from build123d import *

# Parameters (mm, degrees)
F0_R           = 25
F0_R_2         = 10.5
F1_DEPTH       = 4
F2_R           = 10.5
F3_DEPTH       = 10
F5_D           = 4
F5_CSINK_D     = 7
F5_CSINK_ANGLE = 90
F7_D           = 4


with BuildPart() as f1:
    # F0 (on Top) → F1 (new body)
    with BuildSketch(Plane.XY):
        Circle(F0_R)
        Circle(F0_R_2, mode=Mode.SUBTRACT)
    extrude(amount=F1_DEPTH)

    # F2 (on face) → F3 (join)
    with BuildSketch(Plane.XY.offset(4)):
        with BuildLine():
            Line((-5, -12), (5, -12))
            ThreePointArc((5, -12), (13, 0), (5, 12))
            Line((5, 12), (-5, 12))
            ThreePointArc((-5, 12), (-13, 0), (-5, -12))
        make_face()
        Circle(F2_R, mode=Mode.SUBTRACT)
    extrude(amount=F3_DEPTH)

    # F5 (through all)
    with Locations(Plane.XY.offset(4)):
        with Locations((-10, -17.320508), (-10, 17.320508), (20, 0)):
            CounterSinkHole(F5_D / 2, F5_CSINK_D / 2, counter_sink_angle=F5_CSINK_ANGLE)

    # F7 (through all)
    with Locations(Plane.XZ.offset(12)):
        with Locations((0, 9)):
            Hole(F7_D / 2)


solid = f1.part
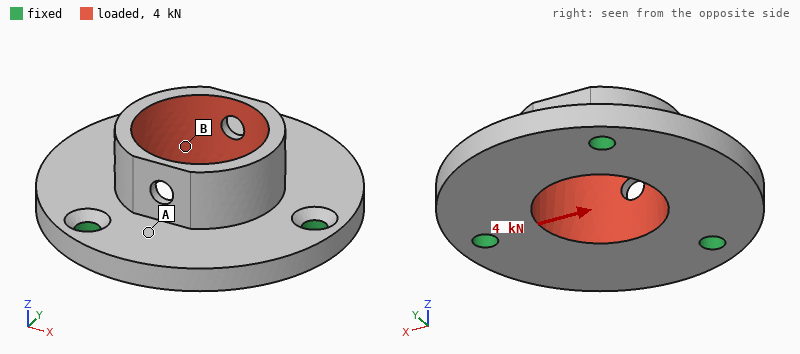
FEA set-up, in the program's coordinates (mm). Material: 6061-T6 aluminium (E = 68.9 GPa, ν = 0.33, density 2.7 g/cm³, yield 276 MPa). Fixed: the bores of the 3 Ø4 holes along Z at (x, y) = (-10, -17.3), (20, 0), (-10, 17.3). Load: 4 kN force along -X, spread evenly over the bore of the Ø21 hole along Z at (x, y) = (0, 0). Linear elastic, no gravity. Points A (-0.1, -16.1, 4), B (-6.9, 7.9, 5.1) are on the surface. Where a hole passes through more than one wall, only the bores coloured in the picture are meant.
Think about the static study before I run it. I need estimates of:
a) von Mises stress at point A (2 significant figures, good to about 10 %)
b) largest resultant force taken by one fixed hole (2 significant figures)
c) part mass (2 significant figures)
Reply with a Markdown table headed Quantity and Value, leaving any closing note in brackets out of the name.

| Quantity | Value |
|---|---|
| von Mises stress at point A | 18 MPa |
| largest resultant force taken by one fixed hole | 1.5 kN |
| part mass | 21 g |
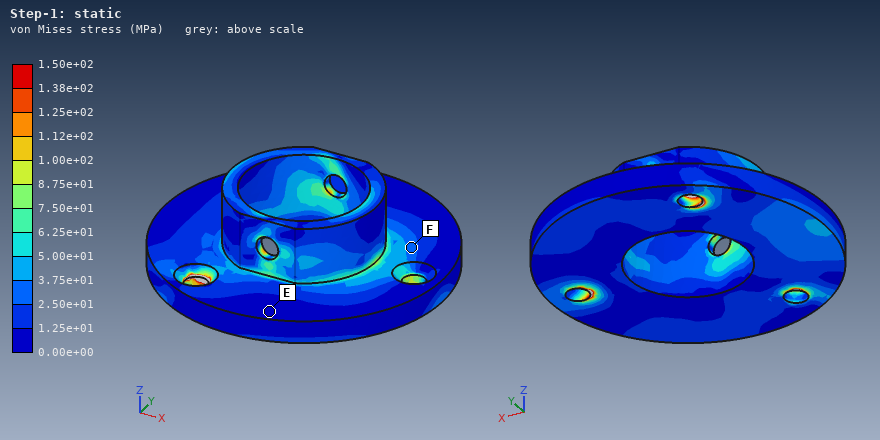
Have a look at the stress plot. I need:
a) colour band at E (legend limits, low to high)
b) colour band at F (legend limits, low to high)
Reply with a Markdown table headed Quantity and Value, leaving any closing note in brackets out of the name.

| Quantity | Value |
|---|---|
| colour band at E | 0.00e+00 to 1.25e+01 MPa |
| colour band at F | 2.50e+01 to 3.75e+01 MPa |
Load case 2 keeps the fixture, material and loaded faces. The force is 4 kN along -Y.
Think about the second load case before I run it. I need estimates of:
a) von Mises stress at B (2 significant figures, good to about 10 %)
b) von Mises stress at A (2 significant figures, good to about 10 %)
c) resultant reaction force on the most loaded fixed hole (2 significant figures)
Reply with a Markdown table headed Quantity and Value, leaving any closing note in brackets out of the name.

| Quantity | Value |
|---|---|
| von Mises stress at B | 41 MPa |
| von Mises stress at A | 32 MPa |
| resultant reaction force on the most loaded fixed hole | 1.4 kN |
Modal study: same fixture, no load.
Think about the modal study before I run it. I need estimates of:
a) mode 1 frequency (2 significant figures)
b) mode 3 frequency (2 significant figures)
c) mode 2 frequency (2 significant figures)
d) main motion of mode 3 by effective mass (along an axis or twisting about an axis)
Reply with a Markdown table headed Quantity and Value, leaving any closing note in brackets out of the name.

| Quantity | Value |
|---|---|
| mode 1 frequency | 9500 Hz |
| mode 3 frequency | 12 kHz |
| mode 2 frequency | 9700 Hz |
| main motion of mode 3 by effective mass | along Z |
